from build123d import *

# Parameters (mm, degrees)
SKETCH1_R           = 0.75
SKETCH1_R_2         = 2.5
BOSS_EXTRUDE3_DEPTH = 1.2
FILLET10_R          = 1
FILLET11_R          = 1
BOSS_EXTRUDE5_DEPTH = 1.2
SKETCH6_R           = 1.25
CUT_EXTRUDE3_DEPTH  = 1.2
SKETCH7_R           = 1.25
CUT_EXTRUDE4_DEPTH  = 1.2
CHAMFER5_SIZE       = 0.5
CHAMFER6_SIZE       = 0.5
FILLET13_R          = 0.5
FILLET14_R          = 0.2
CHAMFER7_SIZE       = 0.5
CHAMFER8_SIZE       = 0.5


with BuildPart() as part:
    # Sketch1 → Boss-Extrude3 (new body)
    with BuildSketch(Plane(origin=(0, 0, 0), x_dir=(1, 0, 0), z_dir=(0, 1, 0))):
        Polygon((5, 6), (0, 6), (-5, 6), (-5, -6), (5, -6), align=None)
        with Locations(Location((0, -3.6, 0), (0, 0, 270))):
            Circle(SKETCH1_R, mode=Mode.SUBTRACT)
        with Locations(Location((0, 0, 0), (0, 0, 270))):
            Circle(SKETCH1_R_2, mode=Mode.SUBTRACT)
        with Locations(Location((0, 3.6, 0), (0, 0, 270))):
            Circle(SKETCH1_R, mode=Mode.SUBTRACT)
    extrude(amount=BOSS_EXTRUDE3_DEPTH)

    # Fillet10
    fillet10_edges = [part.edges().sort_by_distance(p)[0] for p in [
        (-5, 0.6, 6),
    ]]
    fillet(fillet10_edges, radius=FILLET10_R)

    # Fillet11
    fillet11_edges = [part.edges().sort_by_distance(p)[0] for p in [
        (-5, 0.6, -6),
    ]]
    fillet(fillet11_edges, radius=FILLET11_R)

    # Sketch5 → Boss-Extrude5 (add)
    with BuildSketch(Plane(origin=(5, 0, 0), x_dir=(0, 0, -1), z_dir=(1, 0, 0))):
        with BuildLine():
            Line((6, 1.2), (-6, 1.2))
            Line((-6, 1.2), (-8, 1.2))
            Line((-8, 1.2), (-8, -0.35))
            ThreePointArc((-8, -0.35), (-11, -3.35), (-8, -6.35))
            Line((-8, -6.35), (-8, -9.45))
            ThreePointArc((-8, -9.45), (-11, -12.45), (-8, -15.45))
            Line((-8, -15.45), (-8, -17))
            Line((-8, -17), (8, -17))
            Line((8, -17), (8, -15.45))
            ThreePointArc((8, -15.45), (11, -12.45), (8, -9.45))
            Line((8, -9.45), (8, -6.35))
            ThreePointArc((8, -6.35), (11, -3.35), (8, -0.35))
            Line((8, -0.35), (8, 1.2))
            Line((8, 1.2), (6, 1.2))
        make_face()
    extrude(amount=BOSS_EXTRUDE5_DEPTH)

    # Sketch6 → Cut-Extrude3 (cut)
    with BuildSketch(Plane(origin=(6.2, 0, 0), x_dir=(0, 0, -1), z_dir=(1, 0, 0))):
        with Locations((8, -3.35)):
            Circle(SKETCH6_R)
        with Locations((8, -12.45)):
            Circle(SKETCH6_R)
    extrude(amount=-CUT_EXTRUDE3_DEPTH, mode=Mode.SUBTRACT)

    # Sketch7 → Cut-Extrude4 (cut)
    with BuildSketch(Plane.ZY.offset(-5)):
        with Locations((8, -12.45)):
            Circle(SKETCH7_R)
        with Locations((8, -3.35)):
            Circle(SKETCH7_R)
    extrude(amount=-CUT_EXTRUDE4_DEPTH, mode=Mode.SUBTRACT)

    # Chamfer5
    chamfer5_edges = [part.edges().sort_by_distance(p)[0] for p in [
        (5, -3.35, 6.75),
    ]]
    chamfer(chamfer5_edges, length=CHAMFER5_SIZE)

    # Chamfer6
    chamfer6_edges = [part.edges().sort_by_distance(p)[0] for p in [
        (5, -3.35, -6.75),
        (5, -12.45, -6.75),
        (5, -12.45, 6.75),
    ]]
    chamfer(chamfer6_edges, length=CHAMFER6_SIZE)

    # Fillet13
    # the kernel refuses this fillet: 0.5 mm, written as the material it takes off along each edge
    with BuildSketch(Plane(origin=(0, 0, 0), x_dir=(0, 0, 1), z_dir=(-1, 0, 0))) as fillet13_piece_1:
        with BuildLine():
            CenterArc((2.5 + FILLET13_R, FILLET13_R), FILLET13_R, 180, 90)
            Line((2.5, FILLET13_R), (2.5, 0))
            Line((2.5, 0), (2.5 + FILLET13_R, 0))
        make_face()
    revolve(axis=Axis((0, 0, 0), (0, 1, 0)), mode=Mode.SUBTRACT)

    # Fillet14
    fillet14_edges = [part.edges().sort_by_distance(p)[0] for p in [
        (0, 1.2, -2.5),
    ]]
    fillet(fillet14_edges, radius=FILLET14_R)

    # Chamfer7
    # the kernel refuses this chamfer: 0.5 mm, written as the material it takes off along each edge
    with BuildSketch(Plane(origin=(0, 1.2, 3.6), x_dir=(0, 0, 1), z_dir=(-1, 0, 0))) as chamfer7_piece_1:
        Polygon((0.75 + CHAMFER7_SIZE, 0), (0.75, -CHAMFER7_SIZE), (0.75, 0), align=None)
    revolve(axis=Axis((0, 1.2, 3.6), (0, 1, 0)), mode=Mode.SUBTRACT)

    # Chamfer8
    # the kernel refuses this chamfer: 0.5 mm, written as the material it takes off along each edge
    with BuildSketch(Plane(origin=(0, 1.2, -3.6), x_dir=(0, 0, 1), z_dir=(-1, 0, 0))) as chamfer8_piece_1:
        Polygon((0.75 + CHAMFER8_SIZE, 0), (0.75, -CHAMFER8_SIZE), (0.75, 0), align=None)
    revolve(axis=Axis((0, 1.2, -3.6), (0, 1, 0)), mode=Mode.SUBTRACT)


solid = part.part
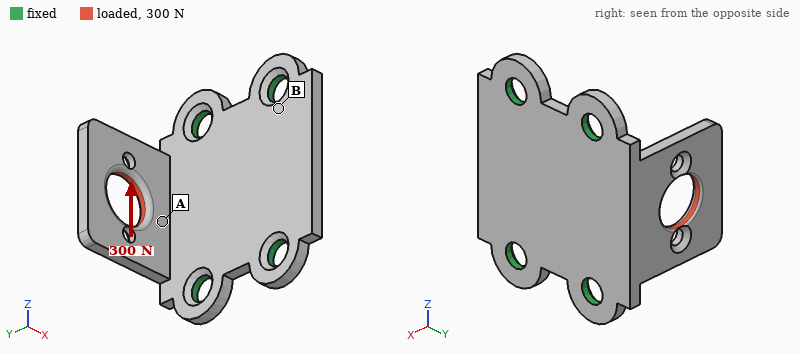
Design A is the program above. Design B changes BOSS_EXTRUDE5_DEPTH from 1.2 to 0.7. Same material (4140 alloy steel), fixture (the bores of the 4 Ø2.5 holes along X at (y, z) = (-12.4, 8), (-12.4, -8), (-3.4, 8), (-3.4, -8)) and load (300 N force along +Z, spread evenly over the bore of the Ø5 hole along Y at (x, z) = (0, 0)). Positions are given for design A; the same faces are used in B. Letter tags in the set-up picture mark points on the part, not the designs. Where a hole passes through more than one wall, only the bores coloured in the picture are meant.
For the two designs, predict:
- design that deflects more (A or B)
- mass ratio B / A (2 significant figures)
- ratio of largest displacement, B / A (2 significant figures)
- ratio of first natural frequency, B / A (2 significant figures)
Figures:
B
0.67
2.8
0.60
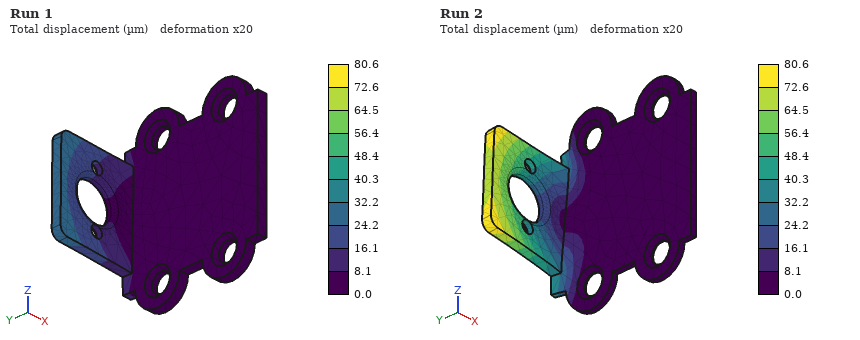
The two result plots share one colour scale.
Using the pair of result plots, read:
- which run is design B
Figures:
Run 2
